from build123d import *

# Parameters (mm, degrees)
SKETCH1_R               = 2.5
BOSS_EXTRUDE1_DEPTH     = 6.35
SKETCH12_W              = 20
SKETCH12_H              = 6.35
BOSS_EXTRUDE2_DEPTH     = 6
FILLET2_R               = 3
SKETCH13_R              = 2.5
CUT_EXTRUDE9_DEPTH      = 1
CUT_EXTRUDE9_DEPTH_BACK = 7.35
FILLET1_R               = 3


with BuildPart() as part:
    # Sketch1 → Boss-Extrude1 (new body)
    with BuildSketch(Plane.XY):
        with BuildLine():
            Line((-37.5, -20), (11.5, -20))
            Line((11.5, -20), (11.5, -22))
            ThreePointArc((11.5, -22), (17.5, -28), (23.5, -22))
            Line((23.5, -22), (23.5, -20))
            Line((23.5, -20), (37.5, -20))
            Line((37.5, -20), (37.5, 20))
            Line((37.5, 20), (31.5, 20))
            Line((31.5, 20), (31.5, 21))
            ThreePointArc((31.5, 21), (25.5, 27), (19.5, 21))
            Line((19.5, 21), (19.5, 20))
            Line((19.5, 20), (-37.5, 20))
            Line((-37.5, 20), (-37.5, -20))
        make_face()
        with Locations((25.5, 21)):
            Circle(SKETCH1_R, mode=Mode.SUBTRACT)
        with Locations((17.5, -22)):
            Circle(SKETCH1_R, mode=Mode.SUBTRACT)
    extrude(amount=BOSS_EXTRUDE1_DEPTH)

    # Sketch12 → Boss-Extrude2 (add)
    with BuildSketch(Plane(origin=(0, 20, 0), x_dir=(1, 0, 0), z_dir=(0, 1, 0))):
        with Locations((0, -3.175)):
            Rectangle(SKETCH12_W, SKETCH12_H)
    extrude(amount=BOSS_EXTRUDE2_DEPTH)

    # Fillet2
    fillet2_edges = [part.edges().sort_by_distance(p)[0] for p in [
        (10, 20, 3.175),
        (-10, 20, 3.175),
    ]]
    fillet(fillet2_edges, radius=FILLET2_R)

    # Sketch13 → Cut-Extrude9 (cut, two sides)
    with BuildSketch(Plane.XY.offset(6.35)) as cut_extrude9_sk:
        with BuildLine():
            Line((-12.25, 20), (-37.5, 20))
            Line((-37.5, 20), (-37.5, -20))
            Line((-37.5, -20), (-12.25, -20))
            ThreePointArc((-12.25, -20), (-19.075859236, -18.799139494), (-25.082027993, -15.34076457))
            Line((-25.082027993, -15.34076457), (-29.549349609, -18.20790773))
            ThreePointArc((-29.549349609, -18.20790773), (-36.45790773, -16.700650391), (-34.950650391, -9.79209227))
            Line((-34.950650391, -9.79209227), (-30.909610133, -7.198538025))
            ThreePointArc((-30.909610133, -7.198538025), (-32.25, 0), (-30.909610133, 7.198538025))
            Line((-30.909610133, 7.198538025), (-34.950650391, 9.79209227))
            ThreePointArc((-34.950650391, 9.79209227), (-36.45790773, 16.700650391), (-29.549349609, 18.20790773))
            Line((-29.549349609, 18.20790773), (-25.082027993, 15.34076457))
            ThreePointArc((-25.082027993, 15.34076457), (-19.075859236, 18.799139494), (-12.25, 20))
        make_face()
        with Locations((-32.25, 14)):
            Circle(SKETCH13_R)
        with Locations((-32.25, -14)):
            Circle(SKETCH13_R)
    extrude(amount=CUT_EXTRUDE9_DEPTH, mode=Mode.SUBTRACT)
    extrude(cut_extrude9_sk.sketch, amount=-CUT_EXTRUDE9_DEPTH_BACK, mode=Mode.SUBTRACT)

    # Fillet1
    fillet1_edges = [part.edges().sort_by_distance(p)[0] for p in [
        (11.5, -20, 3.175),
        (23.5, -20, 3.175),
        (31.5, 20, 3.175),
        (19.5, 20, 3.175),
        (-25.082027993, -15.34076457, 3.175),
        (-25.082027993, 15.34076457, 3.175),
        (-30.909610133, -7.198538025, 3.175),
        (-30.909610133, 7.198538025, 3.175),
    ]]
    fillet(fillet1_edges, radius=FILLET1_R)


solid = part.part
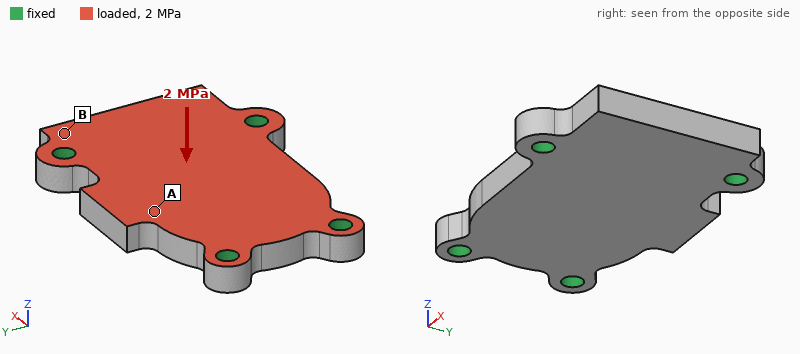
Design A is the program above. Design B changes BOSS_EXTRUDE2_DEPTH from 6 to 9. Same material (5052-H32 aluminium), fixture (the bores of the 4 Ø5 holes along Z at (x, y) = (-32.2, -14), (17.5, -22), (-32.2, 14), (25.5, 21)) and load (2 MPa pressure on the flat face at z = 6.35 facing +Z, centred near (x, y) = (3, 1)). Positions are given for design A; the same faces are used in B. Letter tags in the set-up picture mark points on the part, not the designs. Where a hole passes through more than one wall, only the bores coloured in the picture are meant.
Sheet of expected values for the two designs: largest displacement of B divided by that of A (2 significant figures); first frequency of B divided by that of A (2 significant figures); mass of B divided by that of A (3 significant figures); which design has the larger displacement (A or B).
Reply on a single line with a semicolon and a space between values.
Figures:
1.3; 0.92; 1.02; B
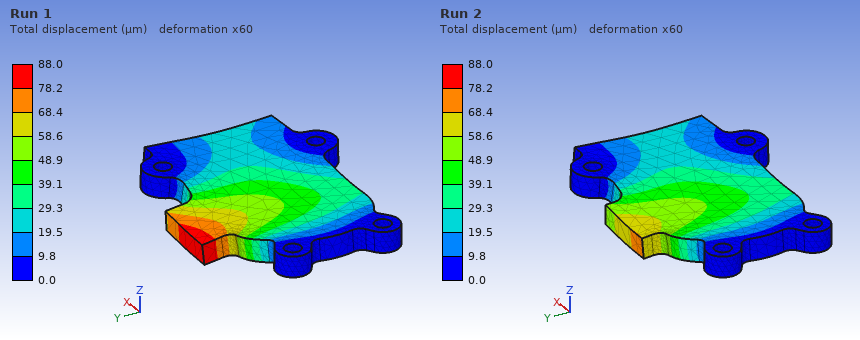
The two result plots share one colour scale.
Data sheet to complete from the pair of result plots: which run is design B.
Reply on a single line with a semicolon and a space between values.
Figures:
Run 1
